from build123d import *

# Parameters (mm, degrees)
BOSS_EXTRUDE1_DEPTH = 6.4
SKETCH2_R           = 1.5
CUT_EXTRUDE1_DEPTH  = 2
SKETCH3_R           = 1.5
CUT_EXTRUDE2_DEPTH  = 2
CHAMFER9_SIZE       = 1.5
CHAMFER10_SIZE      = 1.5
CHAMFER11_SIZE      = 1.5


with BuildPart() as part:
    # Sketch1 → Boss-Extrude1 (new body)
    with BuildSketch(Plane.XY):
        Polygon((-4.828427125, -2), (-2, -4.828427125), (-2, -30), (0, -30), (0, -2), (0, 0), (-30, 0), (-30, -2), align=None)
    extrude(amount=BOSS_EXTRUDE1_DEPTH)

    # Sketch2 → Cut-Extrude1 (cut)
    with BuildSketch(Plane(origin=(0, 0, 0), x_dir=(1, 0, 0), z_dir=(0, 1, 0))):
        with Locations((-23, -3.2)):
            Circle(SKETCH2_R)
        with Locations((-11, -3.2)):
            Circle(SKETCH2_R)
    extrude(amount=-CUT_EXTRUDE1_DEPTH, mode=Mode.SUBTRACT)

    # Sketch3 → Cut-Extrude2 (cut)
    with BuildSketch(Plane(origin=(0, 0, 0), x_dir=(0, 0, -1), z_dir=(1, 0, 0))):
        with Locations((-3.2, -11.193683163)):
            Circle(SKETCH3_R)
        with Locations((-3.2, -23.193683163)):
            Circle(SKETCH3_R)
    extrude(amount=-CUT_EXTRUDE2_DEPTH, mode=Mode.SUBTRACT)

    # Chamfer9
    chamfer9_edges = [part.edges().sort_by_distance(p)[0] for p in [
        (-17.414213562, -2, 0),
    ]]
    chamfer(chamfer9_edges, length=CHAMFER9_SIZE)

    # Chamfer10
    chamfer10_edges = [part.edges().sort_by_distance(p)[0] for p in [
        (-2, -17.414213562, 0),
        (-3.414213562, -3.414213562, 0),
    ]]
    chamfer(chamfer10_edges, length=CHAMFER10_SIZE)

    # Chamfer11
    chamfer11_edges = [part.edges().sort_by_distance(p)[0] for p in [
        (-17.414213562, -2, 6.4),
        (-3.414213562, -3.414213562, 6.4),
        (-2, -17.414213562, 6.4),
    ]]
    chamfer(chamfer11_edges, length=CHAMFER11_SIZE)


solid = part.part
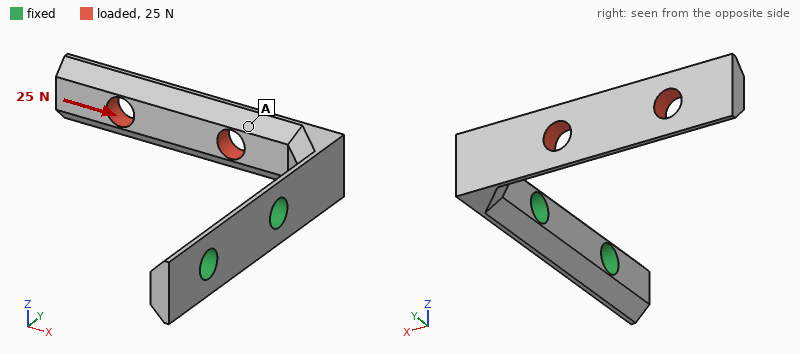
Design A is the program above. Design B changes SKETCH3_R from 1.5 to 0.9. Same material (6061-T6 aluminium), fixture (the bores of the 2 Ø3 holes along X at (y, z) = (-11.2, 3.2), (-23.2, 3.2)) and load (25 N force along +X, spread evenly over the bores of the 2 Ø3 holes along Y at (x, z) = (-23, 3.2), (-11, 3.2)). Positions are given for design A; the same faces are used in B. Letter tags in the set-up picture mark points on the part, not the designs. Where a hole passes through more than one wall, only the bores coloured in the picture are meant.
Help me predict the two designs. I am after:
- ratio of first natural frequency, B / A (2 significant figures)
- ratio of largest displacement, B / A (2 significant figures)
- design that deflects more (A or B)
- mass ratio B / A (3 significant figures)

0.97
1.2
B
1.03
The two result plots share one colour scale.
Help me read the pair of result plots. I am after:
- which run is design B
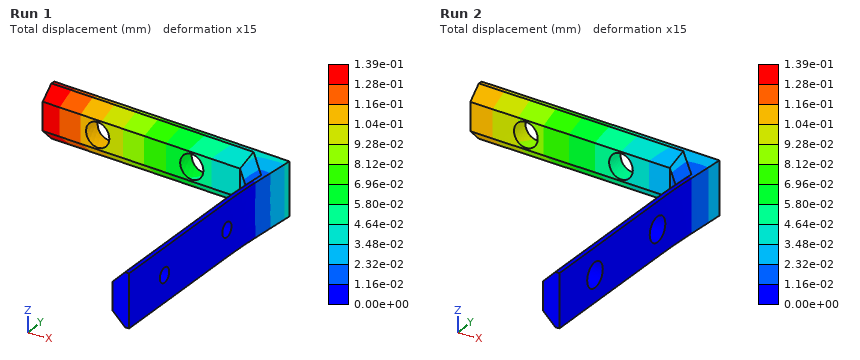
Run 1
